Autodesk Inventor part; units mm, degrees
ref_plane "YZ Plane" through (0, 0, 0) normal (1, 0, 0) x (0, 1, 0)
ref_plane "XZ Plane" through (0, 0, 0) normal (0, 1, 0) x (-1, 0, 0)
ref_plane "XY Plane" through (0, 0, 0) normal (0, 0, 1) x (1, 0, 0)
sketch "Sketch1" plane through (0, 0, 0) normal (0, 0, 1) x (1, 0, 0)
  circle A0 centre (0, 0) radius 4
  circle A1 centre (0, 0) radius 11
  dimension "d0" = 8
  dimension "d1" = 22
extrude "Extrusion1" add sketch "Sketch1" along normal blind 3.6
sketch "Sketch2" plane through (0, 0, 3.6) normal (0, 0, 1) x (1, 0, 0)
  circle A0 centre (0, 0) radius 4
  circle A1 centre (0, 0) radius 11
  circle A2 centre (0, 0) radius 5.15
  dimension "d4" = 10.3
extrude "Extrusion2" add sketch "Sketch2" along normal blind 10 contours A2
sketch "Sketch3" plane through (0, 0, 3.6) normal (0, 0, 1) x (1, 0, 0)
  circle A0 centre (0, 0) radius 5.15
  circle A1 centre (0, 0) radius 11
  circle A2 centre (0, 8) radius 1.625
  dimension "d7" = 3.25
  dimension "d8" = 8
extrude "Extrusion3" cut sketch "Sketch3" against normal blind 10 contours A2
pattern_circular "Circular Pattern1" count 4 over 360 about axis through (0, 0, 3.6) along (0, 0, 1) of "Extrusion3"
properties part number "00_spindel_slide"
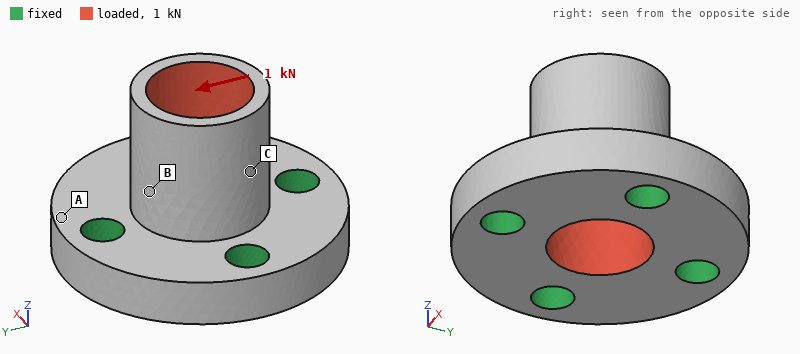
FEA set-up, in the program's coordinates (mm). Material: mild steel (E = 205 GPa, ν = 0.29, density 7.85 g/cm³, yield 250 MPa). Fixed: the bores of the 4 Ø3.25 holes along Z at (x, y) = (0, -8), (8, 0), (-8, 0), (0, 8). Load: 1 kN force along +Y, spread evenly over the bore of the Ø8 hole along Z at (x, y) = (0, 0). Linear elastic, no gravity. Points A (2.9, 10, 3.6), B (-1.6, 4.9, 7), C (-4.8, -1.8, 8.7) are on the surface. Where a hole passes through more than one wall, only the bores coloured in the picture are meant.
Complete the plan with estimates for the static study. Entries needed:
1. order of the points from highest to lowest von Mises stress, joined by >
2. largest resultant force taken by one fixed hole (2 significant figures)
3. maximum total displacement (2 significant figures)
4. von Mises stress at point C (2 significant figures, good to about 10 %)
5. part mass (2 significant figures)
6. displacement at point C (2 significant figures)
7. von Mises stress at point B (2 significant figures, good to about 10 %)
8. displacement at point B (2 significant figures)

C > B > A
450 N
6.2 µm
33 MPa
11 g
3.5 µm
20 MPa
3.1 µm
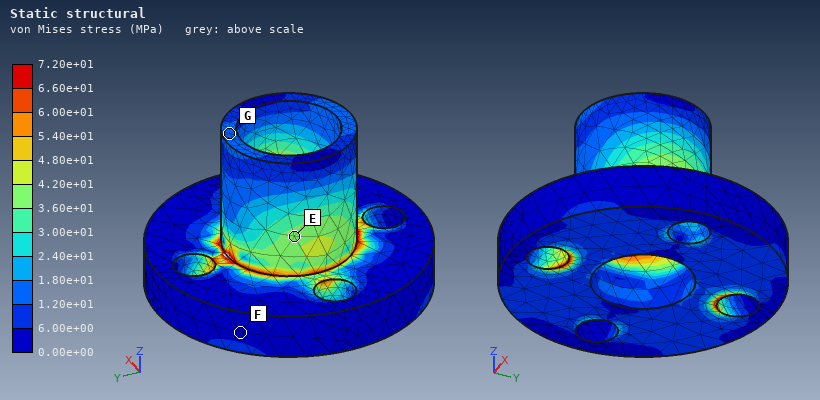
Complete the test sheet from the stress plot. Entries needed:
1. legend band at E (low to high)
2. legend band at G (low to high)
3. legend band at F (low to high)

3.60e+01 to 4.20e+01 MPa
1.20e+01 to 1.80e+01 MPa
0.00e+00 to 6.00e+00 MPa
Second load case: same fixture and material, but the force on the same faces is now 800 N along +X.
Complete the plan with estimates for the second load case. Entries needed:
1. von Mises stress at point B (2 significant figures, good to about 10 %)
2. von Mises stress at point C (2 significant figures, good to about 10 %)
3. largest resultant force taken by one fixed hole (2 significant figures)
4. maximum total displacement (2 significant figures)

32 MPa
15 MPa
360 N
5.0 µm
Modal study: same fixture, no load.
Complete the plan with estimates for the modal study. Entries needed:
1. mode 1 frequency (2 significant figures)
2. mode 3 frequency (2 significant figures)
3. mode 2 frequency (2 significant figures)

40 kHz
43 kHz
40 kHz
